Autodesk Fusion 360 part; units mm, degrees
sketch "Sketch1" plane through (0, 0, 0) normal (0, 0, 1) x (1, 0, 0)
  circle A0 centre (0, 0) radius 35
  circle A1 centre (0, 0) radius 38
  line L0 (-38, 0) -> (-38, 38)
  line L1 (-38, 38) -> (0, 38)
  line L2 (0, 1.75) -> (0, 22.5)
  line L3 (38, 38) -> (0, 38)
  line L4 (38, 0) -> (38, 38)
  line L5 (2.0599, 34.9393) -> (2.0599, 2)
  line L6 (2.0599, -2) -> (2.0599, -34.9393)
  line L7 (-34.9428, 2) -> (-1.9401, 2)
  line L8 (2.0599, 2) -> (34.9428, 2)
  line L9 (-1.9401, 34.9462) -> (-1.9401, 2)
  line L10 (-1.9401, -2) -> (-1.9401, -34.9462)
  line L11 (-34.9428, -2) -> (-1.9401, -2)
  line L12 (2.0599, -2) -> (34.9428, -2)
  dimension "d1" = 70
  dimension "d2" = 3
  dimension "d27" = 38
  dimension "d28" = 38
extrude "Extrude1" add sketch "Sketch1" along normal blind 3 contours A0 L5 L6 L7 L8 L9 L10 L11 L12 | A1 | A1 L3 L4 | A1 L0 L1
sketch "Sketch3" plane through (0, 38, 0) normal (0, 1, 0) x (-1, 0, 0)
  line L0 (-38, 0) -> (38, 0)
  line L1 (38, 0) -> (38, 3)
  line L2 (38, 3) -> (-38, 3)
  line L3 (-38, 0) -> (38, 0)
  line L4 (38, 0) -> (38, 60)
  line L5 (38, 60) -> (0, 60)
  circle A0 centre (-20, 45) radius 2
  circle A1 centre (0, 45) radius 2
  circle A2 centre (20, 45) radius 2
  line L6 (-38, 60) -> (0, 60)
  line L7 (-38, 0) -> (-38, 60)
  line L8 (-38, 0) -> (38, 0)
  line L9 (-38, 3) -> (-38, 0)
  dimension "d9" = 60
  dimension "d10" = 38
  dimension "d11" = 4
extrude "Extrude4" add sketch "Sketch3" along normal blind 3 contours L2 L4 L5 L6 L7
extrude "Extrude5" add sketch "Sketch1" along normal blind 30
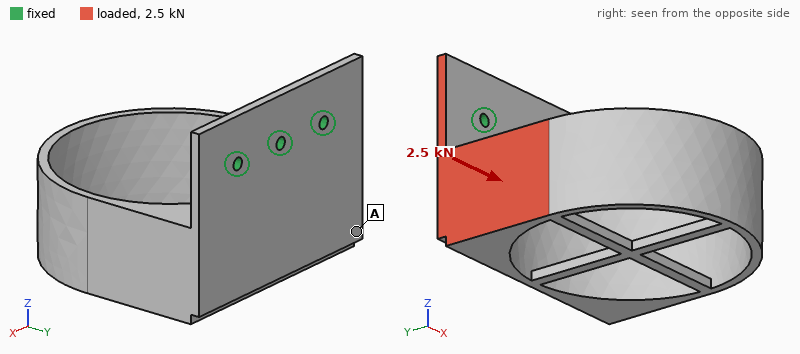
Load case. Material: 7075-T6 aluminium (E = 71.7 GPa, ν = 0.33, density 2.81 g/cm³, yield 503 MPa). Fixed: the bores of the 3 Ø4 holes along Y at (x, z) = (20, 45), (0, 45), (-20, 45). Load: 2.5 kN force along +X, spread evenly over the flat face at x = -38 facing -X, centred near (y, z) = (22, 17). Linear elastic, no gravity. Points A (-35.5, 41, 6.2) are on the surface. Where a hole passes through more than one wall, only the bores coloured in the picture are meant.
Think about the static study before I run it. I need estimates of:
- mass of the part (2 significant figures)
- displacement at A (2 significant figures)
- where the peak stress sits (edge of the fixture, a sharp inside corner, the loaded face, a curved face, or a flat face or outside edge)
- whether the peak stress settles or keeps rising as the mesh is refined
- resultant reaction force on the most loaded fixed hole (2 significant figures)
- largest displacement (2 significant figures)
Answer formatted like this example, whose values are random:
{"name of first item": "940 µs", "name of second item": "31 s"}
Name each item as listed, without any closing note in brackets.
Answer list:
{"mass of the part": "150 g", "displacement at A": "0.27 mm", "where the peak stress sits": "edge of the fixture", "whether the peak stress settles or keeps rising as the mesh is refined": "keeps rising", "resultant reaction force on the most loaded fixed hole": "2.1 kN", "largest displacement": "0.64 mm"}
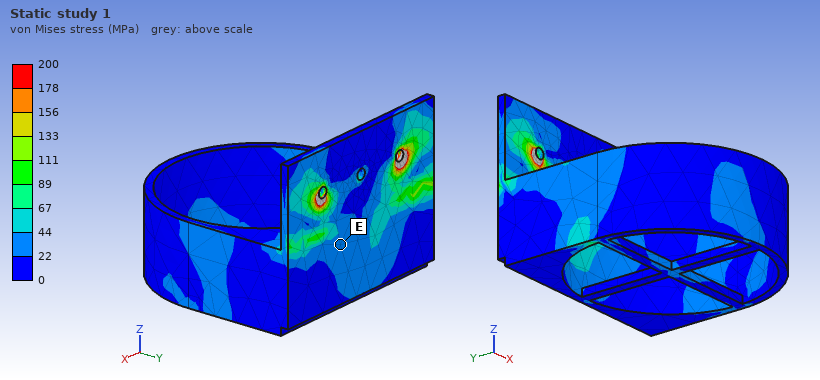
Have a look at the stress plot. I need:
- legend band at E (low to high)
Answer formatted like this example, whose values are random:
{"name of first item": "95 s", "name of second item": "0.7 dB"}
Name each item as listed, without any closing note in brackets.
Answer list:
{"legend band at E": "22 to 44 MPa"}
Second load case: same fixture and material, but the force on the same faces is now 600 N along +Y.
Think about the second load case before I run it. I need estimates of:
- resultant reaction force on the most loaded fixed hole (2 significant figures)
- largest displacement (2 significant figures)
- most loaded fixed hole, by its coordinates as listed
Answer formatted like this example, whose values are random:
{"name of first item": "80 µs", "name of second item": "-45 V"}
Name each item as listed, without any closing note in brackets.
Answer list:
{"resultant reaction force on the most loaded fixed hole": "690 N", "largest displacement": "1.4 mm", "most loaded fixed hole, by its coordinates as listed": "(-20, 45)"}
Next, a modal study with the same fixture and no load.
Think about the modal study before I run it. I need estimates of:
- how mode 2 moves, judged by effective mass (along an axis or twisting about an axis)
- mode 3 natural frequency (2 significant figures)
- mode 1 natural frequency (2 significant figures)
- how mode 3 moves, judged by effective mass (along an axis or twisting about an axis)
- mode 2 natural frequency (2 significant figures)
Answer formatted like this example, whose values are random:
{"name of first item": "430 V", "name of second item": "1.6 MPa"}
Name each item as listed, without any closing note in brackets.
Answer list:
{"how mode 2 moves, judged by effective mass": "along X", "mode 3 natural frequency": "1900 Hz", "mode 1 natural frequency": "290 Hz", "how mode 3 moves, judged by effective mass": "along Y", "mode 2 natural frequency": "760 Hz"}
